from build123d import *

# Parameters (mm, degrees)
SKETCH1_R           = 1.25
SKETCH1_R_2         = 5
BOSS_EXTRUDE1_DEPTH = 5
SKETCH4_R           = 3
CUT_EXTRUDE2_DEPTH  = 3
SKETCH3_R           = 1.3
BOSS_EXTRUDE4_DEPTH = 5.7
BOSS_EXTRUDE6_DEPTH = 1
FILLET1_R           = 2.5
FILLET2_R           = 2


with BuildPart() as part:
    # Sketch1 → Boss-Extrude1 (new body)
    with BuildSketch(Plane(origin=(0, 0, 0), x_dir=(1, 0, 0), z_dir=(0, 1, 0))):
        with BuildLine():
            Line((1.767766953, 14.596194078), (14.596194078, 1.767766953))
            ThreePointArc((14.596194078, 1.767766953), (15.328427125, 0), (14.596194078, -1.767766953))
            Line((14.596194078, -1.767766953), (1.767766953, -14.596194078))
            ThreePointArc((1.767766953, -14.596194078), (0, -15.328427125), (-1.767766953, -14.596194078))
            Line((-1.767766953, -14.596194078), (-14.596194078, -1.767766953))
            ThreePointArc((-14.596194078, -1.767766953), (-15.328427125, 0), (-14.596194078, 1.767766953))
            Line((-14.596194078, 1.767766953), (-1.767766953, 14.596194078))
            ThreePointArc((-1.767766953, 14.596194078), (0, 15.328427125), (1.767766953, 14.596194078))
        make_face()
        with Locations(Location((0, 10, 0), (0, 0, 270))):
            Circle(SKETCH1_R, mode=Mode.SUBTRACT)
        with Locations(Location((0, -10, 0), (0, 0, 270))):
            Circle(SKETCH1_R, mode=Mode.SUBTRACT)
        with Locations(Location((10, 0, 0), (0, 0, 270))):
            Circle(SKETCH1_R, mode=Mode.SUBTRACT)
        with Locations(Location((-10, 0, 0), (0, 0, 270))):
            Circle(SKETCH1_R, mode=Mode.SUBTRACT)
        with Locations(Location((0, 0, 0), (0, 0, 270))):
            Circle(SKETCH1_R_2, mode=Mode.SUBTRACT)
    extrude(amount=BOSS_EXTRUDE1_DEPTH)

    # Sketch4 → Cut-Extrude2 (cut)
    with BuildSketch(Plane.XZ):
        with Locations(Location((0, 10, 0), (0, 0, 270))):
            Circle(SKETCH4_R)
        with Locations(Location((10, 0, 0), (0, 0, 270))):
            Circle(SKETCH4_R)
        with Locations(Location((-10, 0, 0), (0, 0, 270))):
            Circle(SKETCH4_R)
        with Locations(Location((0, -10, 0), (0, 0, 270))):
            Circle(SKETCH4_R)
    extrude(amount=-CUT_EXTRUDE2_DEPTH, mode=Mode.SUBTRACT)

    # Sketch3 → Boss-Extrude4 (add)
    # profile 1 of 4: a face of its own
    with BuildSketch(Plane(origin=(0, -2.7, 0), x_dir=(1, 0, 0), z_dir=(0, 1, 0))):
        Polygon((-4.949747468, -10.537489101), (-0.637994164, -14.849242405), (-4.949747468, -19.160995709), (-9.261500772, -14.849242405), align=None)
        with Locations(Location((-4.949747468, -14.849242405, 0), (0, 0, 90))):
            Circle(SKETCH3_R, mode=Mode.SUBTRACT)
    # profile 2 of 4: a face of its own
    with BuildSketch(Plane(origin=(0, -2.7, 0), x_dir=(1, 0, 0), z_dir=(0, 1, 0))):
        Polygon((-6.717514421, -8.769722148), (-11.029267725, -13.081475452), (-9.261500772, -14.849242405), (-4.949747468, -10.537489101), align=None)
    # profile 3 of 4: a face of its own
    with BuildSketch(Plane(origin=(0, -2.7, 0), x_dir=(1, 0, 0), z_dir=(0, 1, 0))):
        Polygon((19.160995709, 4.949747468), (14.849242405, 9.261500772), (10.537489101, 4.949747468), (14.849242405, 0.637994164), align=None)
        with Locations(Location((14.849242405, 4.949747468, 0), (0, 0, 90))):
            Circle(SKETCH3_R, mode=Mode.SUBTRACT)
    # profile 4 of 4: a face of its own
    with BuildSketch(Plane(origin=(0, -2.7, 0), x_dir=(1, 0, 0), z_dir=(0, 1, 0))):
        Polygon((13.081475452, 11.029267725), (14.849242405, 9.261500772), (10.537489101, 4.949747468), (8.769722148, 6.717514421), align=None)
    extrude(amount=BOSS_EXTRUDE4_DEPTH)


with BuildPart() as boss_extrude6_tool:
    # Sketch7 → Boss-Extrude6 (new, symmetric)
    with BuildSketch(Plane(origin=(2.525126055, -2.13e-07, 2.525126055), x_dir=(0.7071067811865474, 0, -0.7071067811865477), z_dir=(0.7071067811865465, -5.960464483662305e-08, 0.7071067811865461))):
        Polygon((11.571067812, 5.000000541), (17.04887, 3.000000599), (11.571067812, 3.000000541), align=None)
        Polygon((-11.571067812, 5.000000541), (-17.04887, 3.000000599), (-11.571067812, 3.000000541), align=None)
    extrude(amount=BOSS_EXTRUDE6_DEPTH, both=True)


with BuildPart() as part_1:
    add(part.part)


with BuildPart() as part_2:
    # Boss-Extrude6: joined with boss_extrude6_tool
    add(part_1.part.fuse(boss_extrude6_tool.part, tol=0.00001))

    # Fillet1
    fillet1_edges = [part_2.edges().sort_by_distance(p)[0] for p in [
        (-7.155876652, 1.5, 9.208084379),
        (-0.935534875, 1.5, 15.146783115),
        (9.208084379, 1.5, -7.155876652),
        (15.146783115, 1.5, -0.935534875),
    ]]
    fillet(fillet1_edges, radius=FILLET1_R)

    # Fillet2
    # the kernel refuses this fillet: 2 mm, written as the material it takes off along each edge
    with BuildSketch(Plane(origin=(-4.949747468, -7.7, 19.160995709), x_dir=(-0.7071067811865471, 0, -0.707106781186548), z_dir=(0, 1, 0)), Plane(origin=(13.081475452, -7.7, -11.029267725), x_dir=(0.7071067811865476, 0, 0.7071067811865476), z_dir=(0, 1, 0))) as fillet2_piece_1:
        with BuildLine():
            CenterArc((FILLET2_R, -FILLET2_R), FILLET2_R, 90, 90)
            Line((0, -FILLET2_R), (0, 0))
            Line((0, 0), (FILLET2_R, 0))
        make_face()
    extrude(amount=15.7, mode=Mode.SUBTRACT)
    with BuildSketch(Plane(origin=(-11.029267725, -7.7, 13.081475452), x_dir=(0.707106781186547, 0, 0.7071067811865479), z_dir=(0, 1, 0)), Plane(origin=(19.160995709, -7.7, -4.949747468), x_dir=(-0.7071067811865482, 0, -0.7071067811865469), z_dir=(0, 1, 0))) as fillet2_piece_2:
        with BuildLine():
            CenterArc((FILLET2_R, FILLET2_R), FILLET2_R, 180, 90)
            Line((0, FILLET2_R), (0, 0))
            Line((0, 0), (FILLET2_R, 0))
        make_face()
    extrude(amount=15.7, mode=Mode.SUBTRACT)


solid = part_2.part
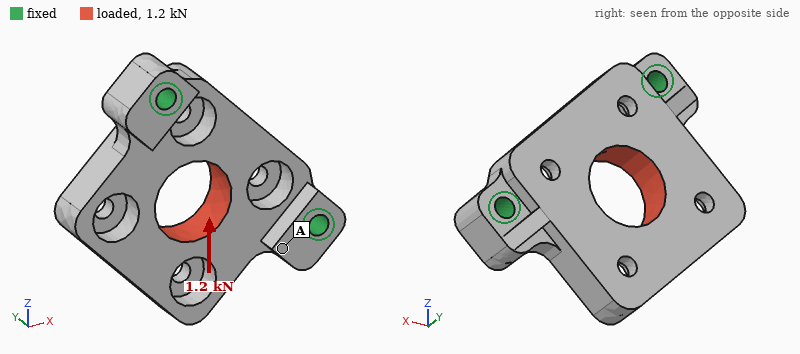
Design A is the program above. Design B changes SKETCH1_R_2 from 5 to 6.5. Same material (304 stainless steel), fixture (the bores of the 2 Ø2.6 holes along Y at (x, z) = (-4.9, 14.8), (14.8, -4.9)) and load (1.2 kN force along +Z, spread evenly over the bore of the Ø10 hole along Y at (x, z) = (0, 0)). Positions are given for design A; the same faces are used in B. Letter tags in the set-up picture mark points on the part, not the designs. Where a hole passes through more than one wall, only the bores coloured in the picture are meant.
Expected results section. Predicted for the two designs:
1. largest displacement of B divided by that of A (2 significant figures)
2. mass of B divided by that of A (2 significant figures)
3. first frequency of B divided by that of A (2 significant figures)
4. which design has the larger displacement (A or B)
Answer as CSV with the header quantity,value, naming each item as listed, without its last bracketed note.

quantity,value
largest displacement of B divided by that of A,1.3
mass of B divided by that of A,0.89
first frequency of B divided by that of A,1.00
which design has the larger displacement,B
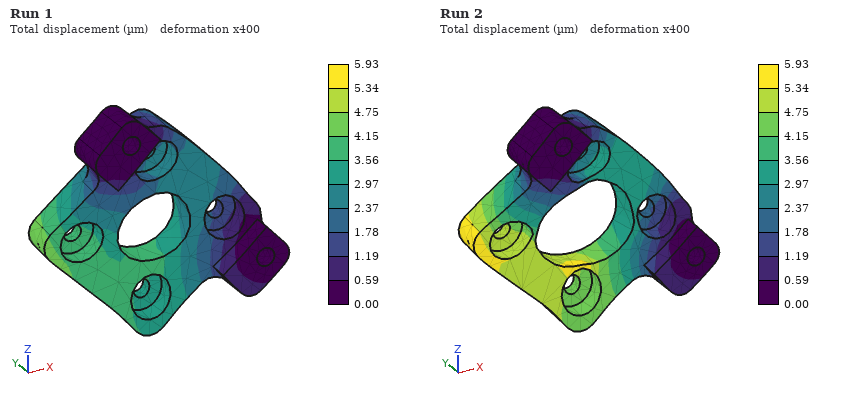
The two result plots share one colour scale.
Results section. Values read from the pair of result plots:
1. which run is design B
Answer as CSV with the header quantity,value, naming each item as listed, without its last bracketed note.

quantity,value
which run is design B,Run 2
